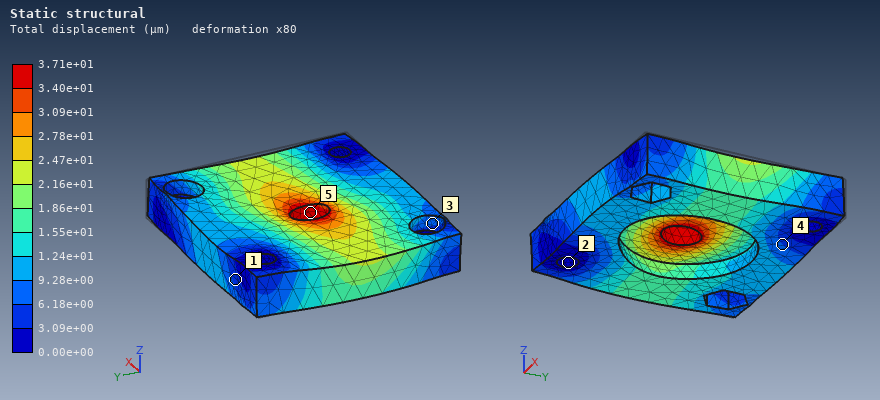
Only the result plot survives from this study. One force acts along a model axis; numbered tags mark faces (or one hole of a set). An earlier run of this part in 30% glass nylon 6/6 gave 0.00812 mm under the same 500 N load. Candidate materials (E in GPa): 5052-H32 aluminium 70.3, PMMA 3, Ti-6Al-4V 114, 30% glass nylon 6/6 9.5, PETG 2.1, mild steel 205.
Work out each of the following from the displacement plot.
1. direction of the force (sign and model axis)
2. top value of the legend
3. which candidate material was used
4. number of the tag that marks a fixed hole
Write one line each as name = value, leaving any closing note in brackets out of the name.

direction of the force = -X
top value of the legend = 3.71e+01 µm
which candidate material was used = PETG
number of the tag that marks a fixed hole = 2
